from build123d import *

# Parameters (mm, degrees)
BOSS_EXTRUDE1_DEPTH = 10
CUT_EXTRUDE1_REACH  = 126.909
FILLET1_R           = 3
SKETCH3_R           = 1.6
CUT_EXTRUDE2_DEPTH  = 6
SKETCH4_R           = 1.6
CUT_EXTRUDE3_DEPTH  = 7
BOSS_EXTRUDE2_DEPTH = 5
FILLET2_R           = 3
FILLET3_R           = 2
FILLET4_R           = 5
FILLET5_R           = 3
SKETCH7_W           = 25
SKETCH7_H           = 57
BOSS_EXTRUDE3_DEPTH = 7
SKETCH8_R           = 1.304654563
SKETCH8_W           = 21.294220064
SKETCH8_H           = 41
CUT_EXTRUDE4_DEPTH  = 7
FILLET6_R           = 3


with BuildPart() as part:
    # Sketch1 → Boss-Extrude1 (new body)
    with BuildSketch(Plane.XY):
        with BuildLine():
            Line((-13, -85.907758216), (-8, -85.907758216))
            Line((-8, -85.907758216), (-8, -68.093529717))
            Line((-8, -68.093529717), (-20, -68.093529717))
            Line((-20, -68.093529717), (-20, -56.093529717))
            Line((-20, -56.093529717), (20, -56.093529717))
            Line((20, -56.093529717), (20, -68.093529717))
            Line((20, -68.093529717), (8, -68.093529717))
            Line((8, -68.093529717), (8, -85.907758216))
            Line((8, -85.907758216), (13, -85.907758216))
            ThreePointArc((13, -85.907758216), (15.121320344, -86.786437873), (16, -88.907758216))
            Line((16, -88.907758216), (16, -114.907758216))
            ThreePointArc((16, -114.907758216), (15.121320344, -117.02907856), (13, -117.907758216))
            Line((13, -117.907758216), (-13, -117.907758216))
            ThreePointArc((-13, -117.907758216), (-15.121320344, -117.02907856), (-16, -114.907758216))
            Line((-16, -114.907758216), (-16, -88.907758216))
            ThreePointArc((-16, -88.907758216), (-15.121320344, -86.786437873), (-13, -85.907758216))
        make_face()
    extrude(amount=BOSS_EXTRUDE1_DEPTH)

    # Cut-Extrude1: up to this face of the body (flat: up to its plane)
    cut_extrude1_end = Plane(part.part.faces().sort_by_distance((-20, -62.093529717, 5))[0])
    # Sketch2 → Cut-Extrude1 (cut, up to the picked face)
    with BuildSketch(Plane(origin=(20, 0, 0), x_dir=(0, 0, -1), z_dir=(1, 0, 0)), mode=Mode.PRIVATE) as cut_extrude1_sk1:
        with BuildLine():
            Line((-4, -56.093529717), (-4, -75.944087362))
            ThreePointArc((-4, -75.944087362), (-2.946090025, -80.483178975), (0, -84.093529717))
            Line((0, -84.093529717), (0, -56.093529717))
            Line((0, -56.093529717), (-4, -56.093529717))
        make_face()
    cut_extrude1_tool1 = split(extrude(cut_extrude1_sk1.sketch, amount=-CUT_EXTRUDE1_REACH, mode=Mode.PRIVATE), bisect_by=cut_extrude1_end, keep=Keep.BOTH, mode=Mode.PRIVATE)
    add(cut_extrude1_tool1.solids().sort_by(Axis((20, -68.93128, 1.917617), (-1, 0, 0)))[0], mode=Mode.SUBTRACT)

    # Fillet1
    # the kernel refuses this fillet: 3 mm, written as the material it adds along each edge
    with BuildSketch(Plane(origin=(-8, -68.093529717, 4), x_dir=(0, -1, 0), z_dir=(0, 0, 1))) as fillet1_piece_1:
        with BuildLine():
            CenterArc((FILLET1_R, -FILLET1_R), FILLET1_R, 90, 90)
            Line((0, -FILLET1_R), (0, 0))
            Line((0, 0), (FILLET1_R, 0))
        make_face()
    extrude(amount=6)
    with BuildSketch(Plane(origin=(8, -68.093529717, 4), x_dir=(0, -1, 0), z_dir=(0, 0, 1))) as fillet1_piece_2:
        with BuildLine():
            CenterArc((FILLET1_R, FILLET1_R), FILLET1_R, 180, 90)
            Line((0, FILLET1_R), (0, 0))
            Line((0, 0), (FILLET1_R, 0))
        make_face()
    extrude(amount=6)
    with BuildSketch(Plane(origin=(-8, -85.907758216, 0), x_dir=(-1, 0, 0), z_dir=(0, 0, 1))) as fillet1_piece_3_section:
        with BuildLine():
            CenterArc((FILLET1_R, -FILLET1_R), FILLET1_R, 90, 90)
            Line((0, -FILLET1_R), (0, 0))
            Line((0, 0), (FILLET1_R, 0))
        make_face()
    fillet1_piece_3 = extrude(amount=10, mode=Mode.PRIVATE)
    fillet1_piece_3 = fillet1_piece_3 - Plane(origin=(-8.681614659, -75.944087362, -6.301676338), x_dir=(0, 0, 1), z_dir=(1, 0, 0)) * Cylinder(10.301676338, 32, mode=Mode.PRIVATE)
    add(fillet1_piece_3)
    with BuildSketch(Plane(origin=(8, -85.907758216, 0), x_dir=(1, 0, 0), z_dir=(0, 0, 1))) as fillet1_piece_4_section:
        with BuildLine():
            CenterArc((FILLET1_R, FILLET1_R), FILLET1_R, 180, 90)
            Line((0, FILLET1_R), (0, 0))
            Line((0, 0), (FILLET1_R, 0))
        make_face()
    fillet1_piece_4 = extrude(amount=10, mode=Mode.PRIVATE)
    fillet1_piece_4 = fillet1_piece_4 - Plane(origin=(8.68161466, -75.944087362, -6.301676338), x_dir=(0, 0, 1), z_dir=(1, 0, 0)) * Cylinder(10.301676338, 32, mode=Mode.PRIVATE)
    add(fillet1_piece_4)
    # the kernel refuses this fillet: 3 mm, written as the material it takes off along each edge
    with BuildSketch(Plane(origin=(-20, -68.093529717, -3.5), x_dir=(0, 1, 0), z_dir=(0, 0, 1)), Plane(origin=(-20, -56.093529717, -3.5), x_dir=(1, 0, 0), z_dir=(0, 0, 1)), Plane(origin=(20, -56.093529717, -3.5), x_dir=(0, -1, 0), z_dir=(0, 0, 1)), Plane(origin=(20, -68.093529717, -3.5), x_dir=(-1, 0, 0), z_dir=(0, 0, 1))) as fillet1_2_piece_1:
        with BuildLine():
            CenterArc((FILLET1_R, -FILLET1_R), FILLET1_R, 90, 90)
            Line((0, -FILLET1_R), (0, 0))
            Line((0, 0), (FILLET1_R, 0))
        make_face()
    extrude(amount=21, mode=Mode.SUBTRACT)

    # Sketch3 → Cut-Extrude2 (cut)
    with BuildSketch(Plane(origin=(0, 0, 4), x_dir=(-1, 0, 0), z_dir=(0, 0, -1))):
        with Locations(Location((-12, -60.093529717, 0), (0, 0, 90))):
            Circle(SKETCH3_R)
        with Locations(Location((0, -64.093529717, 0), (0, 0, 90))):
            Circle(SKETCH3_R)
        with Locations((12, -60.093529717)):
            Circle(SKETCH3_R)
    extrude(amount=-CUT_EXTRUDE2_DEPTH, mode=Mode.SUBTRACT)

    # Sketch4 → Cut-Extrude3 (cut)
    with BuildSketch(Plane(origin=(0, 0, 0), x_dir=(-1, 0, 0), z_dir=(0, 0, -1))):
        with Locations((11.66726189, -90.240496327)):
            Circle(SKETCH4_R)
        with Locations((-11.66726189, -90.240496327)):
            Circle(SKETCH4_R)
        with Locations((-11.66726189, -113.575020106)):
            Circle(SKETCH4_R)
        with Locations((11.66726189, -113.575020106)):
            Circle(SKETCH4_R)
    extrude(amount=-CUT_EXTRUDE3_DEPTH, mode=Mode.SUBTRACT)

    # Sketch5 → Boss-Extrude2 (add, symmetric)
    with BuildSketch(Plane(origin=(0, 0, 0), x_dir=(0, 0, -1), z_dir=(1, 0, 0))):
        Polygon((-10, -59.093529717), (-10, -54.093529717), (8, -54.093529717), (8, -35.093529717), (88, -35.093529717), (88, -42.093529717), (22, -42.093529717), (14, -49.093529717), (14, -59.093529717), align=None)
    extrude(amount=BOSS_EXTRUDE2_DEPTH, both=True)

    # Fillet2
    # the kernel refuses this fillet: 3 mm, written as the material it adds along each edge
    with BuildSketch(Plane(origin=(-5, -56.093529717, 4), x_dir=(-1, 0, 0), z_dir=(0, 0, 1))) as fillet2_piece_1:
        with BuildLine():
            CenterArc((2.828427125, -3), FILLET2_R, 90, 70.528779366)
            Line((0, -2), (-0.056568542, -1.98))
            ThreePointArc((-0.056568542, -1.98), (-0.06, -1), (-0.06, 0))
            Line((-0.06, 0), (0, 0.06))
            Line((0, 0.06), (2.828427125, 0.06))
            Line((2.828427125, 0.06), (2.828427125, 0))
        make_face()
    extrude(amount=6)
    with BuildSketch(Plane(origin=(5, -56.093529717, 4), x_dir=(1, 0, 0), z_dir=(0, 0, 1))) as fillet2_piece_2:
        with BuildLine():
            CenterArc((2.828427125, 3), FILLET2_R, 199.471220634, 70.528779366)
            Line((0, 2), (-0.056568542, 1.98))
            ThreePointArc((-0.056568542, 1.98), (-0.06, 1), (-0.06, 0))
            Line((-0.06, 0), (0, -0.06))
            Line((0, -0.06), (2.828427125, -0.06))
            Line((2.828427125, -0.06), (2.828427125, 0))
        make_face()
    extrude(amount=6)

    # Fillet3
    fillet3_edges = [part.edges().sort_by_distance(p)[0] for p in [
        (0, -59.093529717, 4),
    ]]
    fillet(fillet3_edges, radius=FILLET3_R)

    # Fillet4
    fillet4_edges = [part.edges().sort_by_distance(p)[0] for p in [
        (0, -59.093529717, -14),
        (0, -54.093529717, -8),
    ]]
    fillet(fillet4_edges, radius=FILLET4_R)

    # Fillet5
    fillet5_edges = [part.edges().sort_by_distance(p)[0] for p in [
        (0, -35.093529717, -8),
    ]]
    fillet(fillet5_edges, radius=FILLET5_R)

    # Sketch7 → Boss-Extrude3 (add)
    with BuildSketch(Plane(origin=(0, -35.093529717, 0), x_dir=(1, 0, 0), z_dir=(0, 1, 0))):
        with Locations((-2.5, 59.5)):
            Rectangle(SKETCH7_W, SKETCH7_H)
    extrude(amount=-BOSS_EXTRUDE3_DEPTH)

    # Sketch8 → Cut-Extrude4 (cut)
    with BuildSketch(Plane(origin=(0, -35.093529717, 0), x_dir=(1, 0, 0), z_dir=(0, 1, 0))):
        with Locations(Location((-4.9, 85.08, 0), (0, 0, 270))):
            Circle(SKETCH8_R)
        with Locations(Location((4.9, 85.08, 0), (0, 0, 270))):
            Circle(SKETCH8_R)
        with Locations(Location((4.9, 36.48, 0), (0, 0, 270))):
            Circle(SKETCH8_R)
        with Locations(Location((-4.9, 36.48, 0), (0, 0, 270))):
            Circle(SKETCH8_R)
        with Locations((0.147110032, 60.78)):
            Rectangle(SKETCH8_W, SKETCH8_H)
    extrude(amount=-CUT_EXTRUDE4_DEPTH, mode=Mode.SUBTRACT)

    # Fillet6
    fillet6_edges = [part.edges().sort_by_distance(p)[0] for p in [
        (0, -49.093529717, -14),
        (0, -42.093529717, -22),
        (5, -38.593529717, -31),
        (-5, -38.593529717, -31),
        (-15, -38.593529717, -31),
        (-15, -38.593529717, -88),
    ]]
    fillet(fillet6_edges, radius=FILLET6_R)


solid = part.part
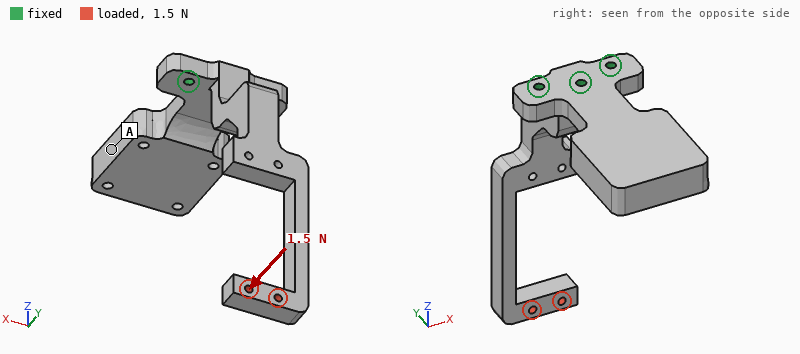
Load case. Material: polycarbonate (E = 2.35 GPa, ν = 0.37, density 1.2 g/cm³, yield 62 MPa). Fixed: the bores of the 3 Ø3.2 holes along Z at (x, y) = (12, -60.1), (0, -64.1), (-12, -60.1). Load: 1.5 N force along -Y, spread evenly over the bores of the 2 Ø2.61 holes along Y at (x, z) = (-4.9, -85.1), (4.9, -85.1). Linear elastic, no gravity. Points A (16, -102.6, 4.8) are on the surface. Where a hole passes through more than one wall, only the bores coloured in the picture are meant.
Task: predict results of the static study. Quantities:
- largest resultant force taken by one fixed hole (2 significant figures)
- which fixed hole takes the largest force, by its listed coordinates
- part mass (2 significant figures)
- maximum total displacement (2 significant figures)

6.6 N
(0, -64.1)
27 g
1.4 mm
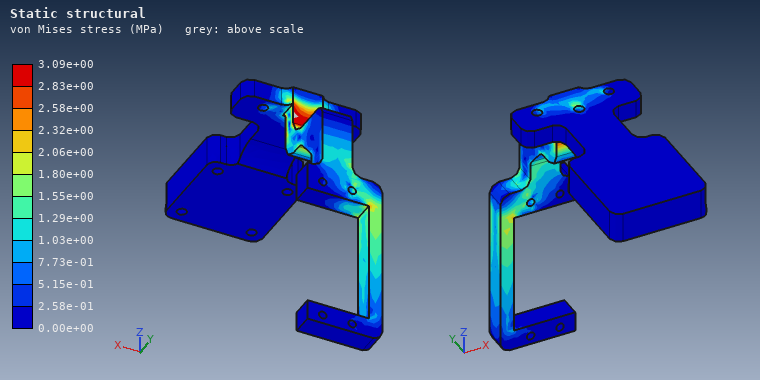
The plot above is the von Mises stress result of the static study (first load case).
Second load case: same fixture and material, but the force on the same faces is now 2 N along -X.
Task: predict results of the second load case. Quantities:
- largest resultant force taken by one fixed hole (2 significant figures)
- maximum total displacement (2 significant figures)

8.9 N
1.3 mm
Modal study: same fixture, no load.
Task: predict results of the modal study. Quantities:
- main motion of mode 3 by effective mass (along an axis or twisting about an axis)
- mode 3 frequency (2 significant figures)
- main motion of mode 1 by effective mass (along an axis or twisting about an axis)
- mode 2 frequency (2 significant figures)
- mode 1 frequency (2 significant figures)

along Z
300 Hz
along Y
150 Hz
120 Hz
